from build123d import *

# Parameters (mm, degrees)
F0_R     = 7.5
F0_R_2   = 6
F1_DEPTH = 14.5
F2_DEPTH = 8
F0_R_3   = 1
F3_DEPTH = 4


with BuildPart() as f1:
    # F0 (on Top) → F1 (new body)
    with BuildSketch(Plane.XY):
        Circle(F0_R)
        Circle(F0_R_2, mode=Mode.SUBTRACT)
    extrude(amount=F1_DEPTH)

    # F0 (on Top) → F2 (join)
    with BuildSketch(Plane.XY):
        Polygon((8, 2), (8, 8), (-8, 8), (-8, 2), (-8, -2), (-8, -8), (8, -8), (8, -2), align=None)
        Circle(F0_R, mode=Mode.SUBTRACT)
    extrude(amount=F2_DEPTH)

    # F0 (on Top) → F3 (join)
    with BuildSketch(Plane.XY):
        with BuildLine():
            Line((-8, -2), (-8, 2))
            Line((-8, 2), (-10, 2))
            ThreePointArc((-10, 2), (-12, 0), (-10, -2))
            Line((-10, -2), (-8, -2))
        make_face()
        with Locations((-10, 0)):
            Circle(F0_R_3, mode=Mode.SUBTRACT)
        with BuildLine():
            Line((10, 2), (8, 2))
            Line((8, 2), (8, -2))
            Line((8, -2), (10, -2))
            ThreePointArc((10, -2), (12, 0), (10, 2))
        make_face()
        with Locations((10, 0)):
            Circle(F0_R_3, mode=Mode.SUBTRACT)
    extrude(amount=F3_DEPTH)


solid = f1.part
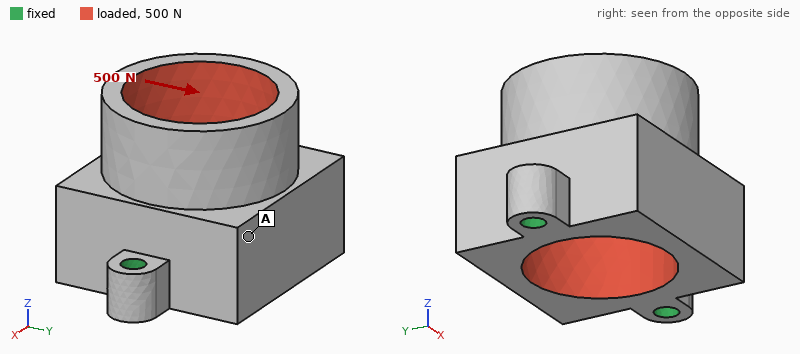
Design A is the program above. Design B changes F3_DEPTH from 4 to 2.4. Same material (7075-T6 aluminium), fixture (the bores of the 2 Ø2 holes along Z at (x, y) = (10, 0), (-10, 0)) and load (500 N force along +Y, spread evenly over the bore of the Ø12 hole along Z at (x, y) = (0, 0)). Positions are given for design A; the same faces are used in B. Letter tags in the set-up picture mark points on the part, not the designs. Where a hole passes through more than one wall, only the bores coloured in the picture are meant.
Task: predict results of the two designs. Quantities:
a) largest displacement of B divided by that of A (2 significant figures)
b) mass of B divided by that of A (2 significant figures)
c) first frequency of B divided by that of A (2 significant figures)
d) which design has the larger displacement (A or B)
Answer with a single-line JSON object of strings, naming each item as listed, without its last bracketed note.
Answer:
{"largest displacement of B divided by that of A": "3.0", "mass of B divided by that of A": "0.98", "first frequency of B divided by that of A": "0.59", "which design has the larger displacement": "B"}
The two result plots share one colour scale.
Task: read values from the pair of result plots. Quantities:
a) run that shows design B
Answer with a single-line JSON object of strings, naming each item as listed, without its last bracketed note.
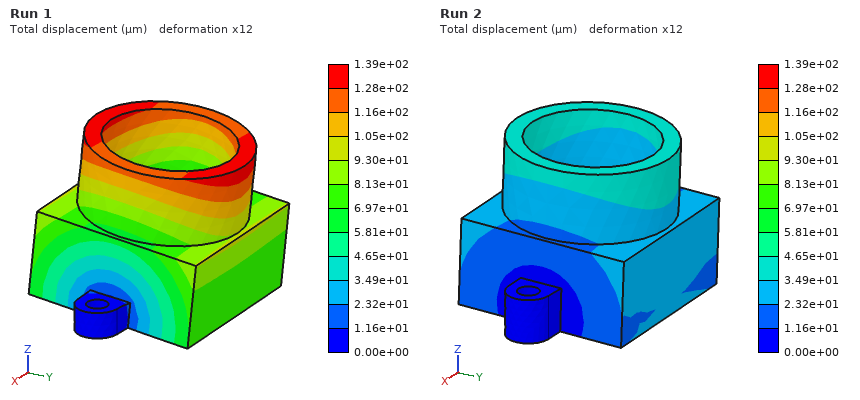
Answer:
{"run that shows design B": "Run 1"}
